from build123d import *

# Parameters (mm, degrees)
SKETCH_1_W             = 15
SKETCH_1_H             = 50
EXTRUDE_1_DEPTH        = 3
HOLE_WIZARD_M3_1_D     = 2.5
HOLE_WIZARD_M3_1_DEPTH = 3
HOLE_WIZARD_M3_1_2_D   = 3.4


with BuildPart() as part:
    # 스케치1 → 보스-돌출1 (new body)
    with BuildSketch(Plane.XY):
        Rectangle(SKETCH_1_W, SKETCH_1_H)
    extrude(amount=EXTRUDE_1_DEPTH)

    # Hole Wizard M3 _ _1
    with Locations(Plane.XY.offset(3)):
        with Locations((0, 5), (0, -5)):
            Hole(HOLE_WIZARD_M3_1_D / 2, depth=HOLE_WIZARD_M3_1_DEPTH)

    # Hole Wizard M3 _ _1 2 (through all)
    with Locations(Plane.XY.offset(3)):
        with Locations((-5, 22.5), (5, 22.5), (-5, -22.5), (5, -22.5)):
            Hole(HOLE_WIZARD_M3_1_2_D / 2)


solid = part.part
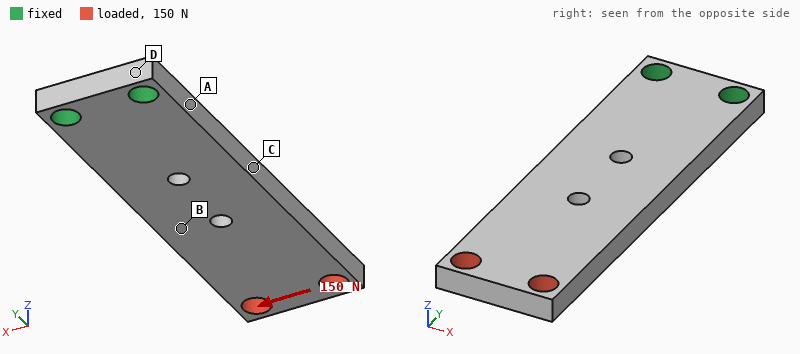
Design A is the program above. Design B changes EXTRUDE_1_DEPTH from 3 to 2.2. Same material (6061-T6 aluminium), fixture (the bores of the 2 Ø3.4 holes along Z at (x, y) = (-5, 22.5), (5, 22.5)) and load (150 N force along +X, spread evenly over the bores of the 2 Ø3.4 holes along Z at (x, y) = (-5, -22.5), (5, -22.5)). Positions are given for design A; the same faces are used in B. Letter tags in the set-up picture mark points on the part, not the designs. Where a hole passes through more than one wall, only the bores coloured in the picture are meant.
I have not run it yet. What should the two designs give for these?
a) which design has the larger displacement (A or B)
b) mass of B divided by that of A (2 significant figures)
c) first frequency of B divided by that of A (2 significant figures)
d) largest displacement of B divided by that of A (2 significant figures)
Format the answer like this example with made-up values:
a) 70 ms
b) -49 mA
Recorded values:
a) B
b) 0.73
c) 0.74
d) 1.4
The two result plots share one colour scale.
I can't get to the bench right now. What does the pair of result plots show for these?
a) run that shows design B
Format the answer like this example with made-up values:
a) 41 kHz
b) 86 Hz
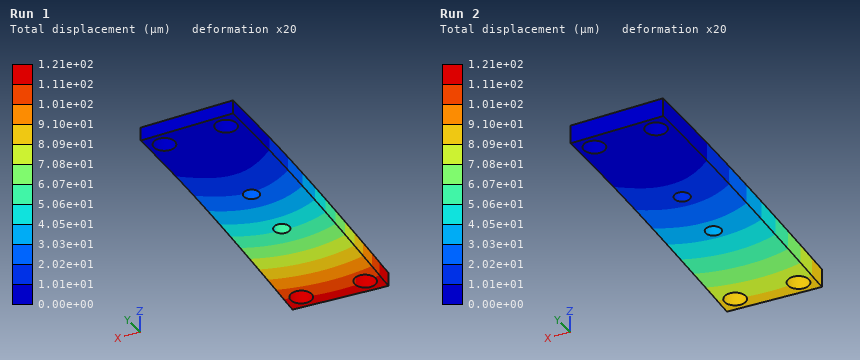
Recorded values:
a) Run 1
